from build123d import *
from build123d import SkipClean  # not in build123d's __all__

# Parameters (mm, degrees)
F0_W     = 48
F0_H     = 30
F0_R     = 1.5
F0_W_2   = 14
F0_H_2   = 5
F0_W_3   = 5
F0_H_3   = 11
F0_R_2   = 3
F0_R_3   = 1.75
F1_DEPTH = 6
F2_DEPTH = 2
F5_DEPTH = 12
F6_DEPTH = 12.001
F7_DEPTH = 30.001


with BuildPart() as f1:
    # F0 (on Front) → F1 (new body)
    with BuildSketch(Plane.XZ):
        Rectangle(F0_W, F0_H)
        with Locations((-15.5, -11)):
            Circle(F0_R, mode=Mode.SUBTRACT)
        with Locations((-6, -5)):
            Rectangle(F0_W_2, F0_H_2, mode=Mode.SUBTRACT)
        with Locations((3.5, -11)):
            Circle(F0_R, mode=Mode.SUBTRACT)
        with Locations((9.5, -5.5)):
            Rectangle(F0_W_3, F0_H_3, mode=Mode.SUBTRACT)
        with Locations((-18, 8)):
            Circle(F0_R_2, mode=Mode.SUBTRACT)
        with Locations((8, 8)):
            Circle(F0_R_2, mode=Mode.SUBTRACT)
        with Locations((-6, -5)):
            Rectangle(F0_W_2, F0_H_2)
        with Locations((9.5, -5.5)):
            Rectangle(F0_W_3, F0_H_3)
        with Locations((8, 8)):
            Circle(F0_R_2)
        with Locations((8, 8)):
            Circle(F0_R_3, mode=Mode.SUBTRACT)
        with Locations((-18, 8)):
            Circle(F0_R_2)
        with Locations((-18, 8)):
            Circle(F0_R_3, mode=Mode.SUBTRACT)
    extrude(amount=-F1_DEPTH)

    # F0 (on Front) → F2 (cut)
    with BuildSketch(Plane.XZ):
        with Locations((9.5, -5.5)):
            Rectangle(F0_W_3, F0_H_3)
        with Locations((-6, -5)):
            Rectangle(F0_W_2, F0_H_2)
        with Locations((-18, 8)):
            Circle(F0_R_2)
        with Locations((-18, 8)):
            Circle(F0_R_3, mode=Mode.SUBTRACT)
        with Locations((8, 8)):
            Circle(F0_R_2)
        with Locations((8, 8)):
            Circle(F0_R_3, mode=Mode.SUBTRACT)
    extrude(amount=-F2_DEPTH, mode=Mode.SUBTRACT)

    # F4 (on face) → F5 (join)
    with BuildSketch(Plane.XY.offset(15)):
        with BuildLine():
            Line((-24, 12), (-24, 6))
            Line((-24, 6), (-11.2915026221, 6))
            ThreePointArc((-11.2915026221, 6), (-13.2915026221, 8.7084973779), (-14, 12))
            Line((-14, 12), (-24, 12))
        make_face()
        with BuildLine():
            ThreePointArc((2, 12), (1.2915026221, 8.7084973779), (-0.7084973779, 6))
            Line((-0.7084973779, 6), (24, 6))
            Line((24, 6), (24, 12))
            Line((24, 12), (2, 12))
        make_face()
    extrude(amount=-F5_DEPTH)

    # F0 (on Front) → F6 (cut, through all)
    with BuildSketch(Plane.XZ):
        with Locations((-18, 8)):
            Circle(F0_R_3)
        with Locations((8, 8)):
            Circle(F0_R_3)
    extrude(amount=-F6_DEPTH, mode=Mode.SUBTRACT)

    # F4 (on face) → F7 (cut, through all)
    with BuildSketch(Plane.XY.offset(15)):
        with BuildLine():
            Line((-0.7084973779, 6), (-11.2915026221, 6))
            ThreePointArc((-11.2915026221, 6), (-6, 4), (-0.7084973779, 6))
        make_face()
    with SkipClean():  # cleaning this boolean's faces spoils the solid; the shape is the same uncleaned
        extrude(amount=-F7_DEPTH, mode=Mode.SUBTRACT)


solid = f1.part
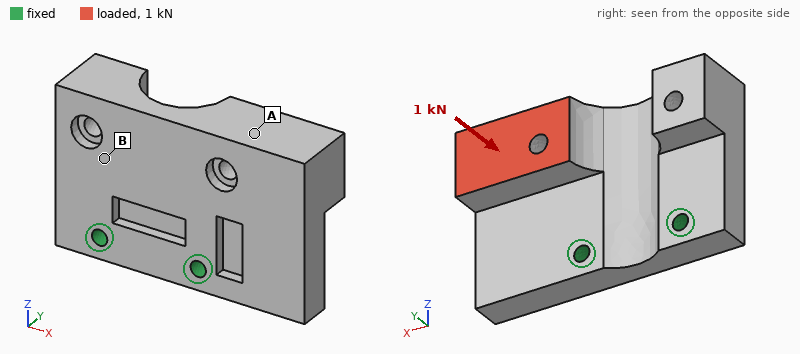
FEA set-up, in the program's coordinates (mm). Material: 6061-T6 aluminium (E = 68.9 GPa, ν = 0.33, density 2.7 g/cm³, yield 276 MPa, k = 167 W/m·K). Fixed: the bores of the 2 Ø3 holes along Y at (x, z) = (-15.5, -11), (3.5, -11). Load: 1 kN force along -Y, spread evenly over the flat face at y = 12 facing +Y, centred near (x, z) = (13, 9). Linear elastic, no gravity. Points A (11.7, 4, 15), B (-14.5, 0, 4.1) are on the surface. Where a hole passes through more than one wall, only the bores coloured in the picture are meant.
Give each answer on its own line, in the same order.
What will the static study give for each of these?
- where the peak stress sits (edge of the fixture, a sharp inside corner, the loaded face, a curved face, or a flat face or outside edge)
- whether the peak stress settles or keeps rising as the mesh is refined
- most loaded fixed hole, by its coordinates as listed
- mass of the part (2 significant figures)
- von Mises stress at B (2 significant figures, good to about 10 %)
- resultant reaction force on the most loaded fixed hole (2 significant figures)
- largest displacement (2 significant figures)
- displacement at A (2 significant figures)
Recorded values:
edge of the fixture
keeps rising
(3.5, -11)
27 g
46 MPa
1.2 kN
0.30 mm
0.22 mm
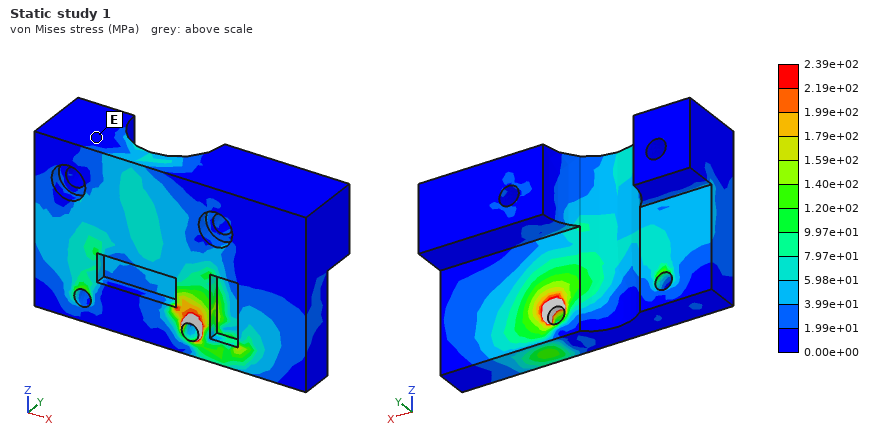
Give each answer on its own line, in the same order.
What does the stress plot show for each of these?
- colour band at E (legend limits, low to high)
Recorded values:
0.00e+00 to 1.99e+01 MPa
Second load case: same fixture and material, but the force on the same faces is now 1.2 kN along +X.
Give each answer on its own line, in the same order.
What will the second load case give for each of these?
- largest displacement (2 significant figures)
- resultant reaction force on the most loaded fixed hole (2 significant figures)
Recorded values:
0.13 mm
1.3 kN
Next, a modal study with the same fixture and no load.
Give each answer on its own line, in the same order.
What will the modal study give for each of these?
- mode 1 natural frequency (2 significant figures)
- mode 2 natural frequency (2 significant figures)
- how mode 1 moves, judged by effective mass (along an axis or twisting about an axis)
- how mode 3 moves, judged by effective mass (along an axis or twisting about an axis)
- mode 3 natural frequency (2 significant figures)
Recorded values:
3500 Hz
5800 Hz
along Y
along X
9500 Hz
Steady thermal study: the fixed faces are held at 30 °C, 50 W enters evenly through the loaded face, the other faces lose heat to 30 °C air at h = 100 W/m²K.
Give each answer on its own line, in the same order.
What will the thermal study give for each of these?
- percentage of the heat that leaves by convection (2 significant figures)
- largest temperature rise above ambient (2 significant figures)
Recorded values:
16 %
46 K
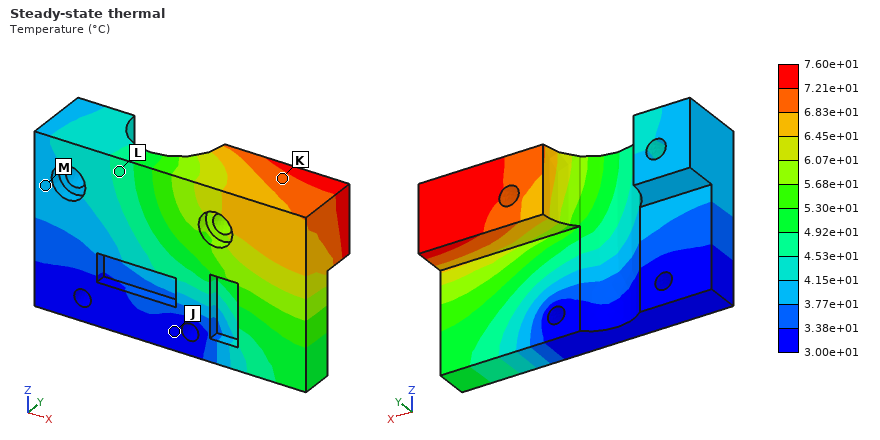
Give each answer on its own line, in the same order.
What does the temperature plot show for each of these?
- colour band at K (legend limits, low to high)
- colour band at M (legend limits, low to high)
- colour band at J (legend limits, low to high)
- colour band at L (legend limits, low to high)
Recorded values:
6.83e+01 to 7.21e+01 °C
3.77e+01 to 4.15e+01 °C
3.00e+01 to 3.38e+01 °C
4.53e+01 to 4.92e+01 °C
